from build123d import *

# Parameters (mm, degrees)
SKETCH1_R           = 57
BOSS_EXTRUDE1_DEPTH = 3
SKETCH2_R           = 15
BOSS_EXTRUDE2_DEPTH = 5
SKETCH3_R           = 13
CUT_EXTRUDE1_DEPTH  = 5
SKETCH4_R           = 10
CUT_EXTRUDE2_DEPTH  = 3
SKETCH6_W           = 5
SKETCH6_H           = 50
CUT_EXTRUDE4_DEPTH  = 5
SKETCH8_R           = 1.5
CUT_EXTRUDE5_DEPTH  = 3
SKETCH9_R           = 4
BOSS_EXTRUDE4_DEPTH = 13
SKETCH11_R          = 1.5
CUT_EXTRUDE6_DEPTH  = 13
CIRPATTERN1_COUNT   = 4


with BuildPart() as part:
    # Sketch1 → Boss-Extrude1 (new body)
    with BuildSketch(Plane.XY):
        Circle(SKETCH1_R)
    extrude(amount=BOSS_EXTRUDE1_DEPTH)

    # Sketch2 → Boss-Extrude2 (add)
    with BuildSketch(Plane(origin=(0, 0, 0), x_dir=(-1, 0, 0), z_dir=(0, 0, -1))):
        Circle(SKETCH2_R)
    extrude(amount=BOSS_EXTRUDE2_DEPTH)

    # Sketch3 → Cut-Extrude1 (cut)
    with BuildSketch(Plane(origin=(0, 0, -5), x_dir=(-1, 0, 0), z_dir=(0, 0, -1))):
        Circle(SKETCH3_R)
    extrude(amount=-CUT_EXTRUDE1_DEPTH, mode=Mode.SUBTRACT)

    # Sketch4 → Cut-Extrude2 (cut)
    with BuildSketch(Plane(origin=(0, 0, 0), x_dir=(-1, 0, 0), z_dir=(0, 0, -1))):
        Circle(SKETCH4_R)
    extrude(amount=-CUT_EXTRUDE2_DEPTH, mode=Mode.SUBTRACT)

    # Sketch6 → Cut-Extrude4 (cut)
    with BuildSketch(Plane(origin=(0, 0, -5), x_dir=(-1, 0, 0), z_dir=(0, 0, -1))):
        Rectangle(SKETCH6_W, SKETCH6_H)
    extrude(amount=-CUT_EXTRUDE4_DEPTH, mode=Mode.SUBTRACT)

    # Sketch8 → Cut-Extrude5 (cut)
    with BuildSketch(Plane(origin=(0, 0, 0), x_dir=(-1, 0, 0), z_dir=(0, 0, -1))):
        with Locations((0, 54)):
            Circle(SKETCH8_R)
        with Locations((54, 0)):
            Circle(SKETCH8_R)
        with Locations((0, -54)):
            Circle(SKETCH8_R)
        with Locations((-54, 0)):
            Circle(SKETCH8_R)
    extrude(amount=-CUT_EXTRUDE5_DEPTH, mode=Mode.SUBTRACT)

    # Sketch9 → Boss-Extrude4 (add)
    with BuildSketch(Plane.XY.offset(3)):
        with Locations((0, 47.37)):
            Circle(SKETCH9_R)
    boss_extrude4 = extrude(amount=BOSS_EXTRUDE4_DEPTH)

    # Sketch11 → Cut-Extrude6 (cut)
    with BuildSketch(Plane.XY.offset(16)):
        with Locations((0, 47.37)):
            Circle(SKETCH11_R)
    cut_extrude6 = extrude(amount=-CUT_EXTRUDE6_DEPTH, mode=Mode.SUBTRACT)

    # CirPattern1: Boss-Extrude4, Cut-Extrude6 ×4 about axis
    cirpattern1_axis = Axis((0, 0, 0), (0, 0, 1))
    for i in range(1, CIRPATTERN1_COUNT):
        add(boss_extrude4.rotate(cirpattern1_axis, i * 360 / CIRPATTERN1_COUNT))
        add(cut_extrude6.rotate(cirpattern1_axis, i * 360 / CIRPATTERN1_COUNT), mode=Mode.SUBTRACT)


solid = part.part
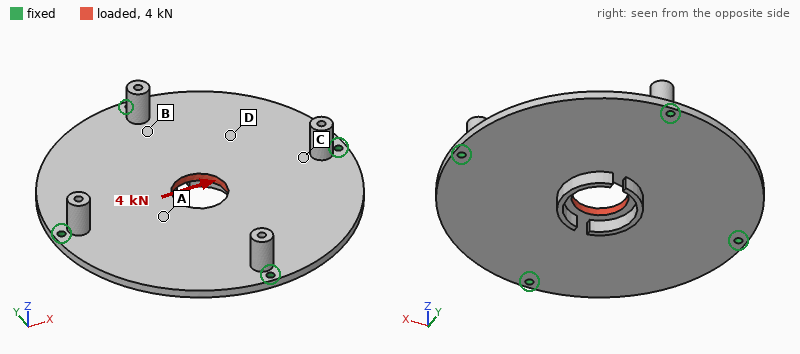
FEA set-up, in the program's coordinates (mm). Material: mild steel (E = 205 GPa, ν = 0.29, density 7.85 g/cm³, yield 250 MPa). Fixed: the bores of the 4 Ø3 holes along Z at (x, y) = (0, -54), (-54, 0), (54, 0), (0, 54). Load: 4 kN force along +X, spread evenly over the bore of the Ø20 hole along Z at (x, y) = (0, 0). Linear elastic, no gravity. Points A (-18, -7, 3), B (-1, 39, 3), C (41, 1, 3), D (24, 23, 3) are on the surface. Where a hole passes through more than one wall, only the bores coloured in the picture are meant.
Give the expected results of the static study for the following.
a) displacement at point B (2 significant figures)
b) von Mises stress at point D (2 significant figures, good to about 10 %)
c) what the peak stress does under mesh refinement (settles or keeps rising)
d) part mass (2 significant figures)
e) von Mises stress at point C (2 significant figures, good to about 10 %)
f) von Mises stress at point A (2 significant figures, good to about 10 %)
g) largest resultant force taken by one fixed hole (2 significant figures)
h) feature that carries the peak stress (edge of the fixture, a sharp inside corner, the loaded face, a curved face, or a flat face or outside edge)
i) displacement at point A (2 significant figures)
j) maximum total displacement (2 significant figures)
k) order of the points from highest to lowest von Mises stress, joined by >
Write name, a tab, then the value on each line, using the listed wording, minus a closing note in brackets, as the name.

displacement at point B	2.0 µm
von Mises stress at point D	6.9 MPa
what the peak stress does under mesh refinement	keeps rising
part mass	260 g
von Mises stress at point C	26 MPa
von Mises stress at point A	20 MPa
largest resultant force taken by one fixed hole	1.2 kN
feature that carries the peak stress	edge of the fixture
displacement at point A	4.0 µm
maximum total displacement	5.2 µm
order of the points from highest to lowest von Mises stress, joined by >	C > A > D > B
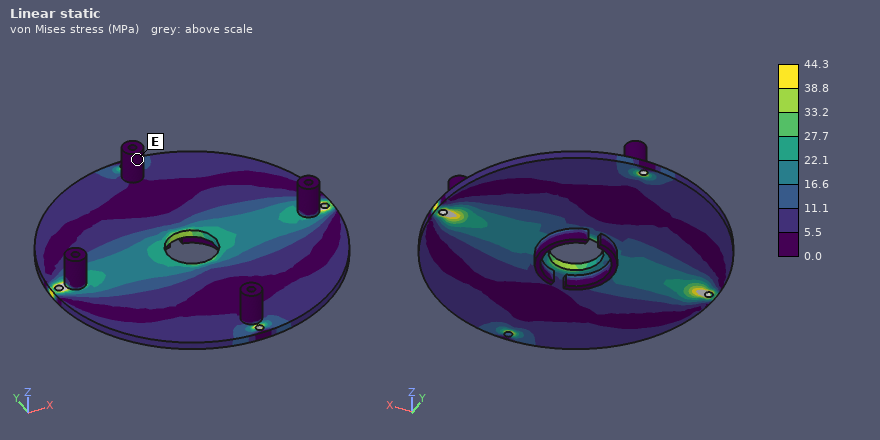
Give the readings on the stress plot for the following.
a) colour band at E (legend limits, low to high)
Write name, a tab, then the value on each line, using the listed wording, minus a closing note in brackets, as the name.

colour band at E	0.0 to 5.5 MPa
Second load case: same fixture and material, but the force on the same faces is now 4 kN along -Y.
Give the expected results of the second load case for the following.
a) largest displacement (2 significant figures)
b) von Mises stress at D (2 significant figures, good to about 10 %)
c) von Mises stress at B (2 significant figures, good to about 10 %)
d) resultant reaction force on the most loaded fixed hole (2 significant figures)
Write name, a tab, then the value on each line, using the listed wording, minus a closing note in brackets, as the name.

largest displacement	5.2 µm
von Mises stress at D	6.8 MPa
von Mises stress at B	24 MPa
resultant reaction force on the most loaded fixed hole	1.2 kN
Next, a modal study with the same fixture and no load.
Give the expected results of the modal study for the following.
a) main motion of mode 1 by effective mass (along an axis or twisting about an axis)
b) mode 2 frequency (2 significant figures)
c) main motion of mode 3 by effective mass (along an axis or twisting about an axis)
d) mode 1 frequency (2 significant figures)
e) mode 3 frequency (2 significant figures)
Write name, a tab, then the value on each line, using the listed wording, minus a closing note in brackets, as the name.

main motion of mode 1 by effective mass	along Z
mode 2 frequency	2300 Hz
main motion of mode 3 by effective mass	twisting about Y
mode 1 frequency	1800 Hz
mode 3 frequency	2400 Hz
